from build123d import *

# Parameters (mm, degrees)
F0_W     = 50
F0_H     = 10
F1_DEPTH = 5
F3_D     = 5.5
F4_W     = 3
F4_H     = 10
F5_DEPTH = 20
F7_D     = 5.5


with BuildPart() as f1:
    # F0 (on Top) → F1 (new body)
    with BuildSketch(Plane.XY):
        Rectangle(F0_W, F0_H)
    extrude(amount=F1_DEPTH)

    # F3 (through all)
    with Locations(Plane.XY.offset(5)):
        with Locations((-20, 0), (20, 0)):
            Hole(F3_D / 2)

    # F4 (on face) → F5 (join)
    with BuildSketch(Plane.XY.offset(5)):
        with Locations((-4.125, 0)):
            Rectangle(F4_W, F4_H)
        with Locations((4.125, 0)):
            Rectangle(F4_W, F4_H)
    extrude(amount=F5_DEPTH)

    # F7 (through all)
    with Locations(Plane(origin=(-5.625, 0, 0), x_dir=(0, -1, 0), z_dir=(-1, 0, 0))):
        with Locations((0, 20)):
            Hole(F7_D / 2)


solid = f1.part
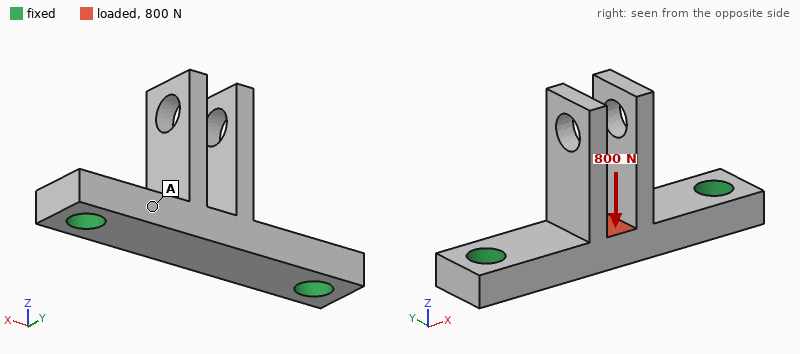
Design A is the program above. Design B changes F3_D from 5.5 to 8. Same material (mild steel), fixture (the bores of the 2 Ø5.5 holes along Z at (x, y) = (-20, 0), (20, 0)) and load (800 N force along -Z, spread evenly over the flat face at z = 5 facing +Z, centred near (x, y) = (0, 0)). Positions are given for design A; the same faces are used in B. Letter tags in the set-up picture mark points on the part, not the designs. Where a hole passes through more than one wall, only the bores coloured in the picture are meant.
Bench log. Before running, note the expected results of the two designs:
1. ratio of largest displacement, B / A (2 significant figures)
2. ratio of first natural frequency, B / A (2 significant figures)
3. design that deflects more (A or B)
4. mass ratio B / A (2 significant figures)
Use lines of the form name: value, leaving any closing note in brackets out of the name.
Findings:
ratio of largest displacement, B / A: 0.87
ratio of first natural frequency, B / A: 1.0
design that deflects more: A
mass ratio B / A: 0.92
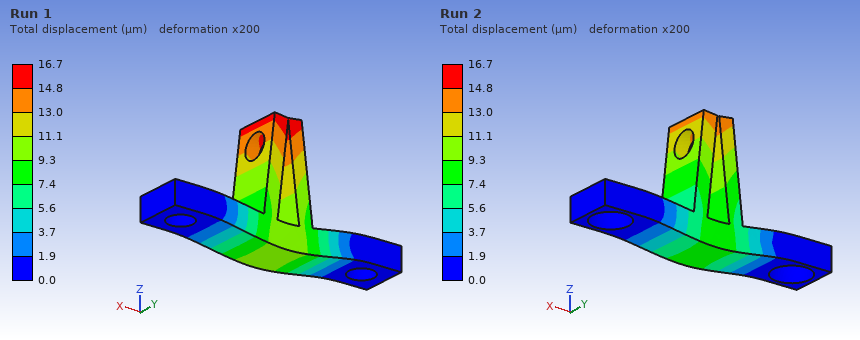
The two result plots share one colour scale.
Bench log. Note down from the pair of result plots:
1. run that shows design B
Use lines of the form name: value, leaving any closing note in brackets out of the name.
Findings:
run that shows design B: Run 2
